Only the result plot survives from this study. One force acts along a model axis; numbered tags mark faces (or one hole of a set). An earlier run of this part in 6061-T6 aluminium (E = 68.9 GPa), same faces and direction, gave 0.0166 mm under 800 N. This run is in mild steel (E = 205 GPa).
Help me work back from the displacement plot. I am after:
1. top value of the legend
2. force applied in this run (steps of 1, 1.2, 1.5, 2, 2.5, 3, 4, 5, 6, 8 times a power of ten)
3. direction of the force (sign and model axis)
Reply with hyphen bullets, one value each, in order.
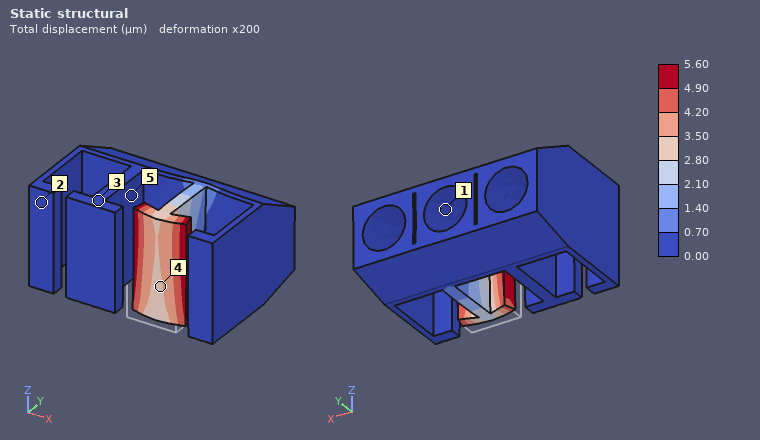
- 5.60 µm
- 800 N
- +Y
